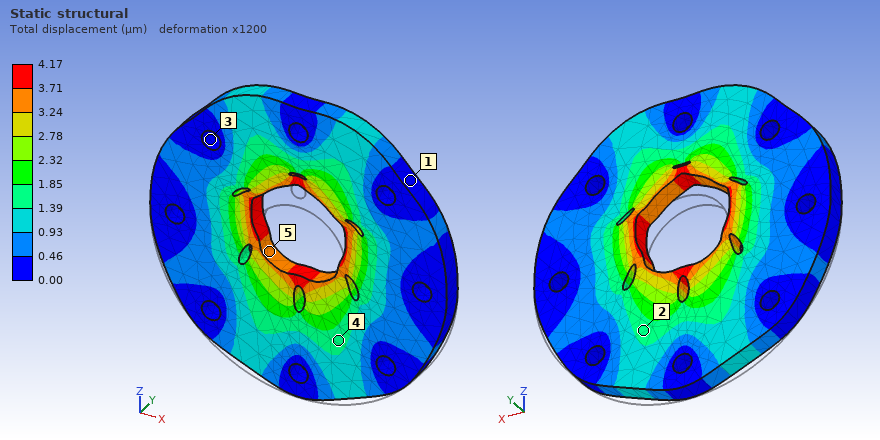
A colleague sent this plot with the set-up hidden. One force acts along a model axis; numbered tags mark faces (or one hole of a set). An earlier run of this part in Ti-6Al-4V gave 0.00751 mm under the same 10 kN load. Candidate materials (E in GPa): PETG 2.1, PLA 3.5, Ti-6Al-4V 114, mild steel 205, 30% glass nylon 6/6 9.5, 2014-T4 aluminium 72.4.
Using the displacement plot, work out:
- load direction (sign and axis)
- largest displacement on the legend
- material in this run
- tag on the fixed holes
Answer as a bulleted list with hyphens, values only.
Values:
- +Z
- 4.17 µm
- mild steel
- 3
